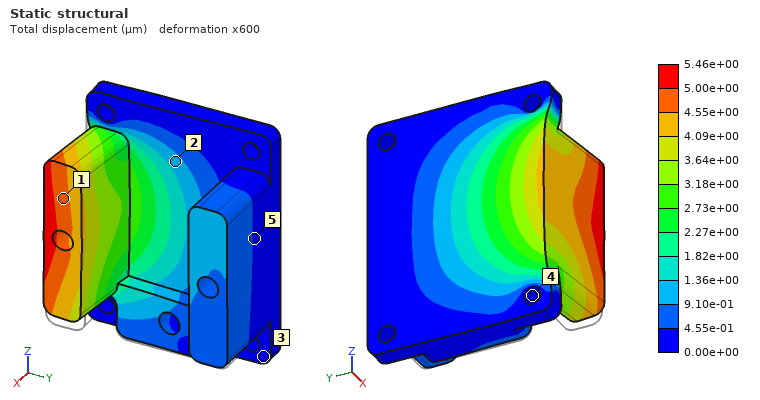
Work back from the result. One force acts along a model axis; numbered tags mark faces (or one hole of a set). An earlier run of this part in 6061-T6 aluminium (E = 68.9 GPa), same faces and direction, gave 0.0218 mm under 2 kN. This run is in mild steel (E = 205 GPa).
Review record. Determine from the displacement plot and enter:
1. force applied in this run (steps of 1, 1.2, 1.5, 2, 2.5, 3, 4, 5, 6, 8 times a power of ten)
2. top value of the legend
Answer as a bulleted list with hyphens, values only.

- 1.5 kN
- 5.46e+00 µm
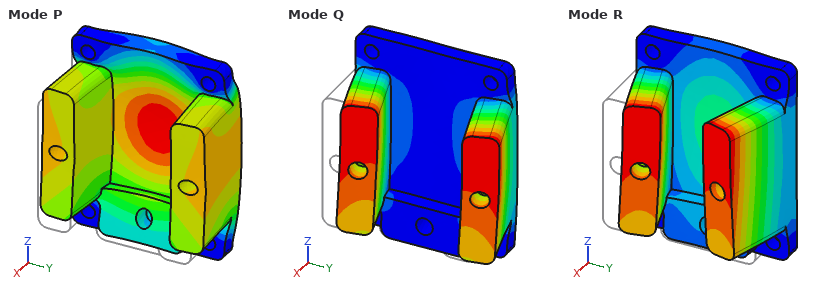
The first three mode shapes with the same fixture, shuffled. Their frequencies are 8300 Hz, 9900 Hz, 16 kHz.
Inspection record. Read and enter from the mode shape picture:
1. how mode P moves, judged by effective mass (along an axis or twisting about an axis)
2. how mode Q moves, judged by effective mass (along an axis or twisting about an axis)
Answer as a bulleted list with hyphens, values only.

- along X
- along Y
